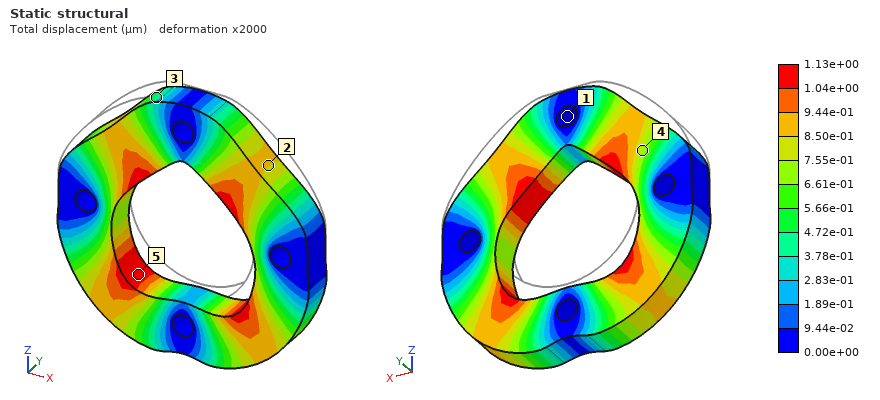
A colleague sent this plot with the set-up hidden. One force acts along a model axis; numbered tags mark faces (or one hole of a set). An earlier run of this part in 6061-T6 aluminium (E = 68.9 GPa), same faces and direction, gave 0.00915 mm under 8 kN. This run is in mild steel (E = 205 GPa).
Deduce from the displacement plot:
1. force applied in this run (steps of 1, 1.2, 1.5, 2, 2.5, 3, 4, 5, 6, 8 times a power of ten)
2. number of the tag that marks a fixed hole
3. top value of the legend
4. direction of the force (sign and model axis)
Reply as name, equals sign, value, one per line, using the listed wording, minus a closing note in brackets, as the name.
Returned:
force applied in this run = 3 kN
number of the tag that marks a fixed hole = 1
top value of the legend = 1.13e+00 µm
direction of the force = -Z
